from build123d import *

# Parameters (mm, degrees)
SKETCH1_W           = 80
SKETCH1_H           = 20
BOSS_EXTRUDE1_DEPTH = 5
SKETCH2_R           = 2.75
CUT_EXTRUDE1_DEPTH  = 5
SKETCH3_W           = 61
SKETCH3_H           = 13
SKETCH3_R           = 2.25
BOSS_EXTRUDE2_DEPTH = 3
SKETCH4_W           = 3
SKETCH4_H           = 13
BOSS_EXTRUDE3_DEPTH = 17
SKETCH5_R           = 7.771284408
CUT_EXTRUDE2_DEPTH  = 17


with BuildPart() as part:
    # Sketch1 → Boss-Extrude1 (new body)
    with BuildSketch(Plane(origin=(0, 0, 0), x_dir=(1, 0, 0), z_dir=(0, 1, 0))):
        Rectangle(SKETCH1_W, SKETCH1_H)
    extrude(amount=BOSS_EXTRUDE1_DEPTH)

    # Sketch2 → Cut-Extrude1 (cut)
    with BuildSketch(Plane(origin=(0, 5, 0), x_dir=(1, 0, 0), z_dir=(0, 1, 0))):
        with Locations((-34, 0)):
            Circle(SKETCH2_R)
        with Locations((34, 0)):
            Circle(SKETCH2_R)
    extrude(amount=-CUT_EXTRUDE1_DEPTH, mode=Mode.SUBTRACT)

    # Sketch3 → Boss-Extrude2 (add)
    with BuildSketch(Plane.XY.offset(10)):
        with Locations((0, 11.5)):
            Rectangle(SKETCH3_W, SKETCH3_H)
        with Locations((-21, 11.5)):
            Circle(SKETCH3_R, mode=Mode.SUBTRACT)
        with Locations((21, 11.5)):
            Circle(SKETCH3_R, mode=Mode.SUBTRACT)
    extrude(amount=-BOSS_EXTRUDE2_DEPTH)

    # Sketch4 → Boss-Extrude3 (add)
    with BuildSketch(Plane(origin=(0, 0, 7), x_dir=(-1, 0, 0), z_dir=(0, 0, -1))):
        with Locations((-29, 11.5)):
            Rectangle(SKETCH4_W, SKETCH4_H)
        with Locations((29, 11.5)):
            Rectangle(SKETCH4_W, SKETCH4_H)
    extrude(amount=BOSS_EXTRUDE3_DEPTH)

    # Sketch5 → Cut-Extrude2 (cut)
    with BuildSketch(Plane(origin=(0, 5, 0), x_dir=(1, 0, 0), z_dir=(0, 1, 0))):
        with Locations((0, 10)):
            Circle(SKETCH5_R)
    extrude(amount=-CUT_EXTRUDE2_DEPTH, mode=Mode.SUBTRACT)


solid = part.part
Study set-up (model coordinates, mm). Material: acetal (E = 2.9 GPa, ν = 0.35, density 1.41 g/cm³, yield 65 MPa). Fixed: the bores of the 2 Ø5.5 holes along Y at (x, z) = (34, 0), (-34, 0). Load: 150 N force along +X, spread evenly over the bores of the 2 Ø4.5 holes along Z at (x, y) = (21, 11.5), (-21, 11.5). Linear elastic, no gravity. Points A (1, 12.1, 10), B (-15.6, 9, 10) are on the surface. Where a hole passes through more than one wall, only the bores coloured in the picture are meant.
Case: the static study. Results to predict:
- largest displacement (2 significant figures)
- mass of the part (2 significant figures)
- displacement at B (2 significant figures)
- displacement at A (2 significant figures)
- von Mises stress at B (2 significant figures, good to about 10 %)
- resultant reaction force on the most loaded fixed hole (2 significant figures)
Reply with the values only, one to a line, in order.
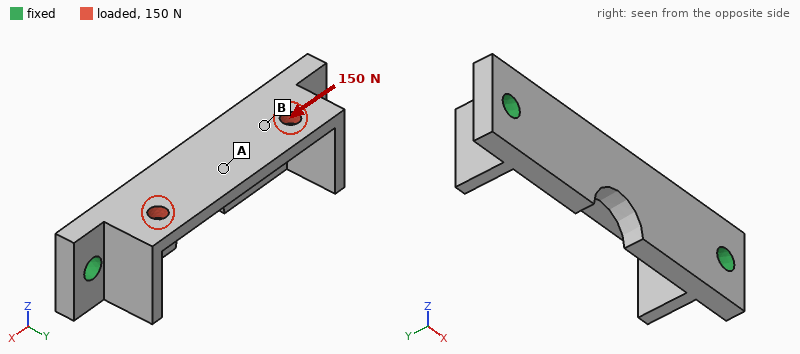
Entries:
22 µm
15 g
11 µm
10 µm
1.3 MPa
80 N
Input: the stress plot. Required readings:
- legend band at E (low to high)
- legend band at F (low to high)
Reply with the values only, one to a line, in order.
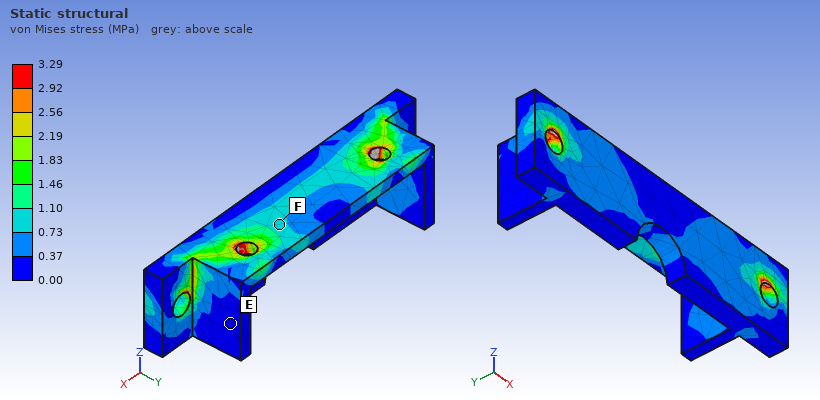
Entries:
0.00 to 0.37 MPa
0.73 to 1.10 MPa
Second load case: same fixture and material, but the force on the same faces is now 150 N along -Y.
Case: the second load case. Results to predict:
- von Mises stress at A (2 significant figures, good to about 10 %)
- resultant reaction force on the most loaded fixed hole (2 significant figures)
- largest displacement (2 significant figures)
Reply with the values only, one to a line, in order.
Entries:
1.2 MPa
80 N
0.11 mm
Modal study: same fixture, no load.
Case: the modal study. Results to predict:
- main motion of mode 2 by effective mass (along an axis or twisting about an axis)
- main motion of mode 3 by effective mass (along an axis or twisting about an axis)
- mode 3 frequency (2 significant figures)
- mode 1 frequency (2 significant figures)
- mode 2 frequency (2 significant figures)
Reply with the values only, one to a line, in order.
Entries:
along Y
along Z
3400 Hz
2100 Hz
2300 Hz
